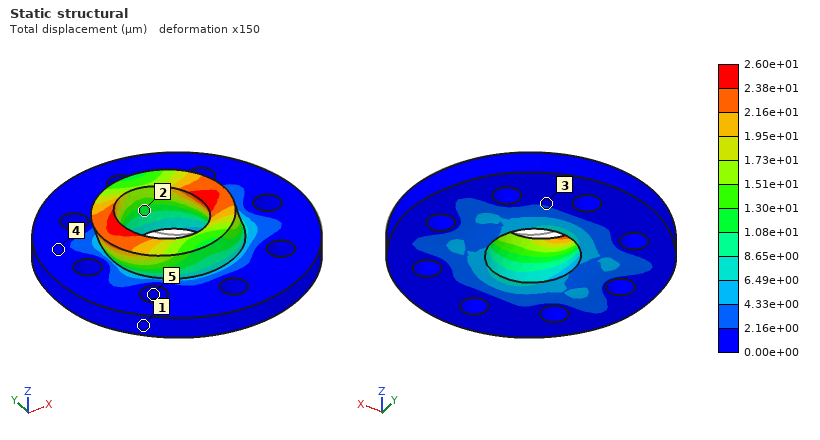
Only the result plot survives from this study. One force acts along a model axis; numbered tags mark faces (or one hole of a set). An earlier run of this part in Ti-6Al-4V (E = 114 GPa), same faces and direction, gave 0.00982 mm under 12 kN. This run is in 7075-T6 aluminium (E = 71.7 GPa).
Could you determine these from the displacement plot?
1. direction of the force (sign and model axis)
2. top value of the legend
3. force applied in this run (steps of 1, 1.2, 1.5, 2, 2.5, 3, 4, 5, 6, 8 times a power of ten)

-X
2.60e+01 µm
20 kN
